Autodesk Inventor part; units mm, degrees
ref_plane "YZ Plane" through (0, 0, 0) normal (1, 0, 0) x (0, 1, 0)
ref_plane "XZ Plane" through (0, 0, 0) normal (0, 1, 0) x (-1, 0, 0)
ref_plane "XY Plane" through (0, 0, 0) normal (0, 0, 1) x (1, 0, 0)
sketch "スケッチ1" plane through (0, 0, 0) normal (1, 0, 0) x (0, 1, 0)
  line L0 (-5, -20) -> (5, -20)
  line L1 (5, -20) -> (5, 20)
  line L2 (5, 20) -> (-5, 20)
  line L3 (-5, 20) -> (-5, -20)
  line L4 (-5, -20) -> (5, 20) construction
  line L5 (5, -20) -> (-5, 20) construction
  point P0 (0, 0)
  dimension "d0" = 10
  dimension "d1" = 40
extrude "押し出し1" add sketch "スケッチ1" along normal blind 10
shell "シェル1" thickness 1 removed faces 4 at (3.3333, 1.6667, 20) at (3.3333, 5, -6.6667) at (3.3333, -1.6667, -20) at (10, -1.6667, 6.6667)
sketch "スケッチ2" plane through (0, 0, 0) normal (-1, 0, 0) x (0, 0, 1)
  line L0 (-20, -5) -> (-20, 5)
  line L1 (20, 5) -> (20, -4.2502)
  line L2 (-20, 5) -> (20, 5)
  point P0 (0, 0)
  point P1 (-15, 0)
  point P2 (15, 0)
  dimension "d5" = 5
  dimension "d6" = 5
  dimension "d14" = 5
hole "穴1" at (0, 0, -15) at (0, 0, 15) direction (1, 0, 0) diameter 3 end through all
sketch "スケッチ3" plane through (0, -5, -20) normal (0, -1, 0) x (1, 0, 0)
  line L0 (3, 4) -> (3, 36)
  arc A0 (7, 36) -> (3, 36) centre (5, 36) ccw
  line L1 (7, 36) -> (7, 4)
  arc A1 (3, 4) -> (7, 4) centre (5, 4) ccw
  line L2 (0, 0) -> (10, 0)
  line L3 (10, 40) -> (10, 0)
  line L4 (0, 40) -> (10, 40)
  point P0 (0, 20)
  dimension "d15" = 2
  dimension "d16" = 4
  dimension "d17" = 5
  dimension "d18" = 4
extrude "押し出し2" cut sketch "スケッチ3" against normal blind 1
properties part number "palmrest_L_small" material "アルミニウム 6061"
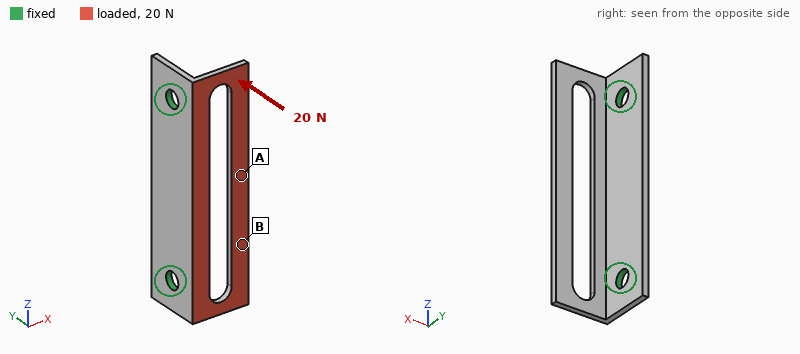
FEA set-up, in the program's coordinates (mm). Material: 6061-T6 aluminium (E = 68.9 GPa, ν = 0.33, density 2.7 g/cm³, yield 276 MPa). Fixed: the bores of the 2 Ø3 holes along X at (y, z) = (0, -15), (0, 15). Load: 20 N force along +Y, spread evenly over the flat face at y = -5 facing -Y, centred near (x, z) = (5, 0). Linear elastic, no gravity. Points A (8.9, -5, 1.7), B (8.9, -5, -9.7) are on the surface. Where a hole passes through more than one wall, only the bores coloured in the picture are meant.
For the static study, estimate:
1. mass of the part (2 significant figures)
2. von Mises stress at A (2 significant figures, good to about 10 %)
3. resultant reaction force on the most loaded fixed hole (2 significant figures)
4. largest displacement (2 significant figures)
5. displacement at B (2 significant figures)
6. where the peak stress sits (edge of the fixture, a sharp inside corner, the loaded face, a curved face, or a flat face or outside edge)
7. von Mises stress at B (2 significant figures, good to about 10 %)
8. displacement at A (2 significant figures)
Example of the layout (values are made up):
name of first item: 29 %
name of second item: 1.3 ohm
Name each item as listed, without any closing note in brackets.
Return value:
mass of the part: 1.6 g
von Mises stress at A: 39 MPa
resultant reaction force on the most loaded fixed hole: 10 N
largest displacement: 0.22 mm
displacement at B: 0.15 mm
where the peak stress sits: a flat face or outside edge
von Mises stress at B: 18 MPa
displacement at A: 0.20 mm
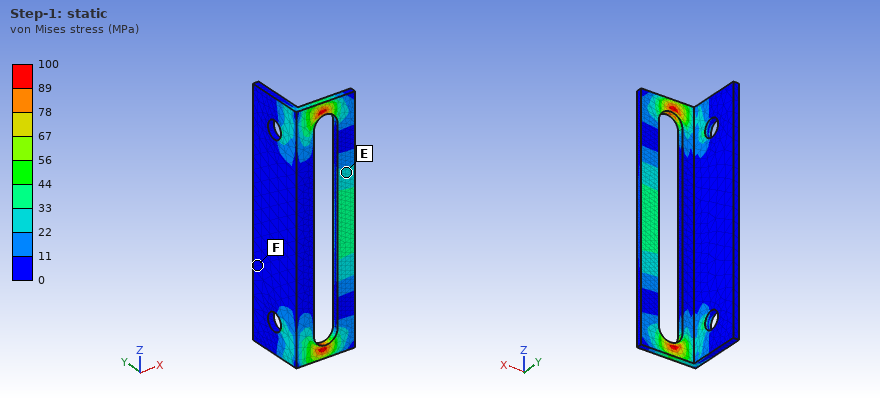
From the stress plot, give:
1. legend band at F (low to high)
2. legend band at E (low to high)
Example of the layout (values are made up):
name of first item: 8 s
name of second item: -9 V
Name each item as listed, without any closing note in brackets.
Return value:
legend band at F: 0 to 11 MPa
legend band at E: 22 to 33 MPa
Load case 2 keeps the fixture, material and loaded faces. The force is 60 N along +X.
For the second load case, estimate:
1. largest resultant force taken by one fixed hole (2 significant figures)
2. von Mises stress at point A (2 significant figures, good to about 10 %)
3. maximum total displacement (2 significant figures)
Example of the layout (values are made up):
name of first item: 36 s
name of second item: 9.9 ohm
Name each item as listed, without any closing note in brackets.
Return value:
largest resultant force taken by one fixed hole: 30 N
von Mises stress at point A: 12 MPa
maximum total displacement: 85 µm
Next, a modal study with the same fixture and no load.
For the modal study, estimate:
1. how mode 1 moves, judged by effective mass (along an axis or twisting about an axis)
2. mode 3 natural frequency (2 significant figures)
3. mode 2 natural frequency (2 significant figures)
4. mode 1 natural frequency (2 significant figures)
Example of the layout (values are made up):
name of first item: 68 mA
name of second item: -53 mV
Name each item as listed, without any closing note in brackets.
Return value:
how mode 1 moves, judged by effective mass: along Y
mode 3 natural frequency: 6500 Hz
mode 2 natural frequency: 5100 Hz
mode 1 natural frequency: 2200 Hz
